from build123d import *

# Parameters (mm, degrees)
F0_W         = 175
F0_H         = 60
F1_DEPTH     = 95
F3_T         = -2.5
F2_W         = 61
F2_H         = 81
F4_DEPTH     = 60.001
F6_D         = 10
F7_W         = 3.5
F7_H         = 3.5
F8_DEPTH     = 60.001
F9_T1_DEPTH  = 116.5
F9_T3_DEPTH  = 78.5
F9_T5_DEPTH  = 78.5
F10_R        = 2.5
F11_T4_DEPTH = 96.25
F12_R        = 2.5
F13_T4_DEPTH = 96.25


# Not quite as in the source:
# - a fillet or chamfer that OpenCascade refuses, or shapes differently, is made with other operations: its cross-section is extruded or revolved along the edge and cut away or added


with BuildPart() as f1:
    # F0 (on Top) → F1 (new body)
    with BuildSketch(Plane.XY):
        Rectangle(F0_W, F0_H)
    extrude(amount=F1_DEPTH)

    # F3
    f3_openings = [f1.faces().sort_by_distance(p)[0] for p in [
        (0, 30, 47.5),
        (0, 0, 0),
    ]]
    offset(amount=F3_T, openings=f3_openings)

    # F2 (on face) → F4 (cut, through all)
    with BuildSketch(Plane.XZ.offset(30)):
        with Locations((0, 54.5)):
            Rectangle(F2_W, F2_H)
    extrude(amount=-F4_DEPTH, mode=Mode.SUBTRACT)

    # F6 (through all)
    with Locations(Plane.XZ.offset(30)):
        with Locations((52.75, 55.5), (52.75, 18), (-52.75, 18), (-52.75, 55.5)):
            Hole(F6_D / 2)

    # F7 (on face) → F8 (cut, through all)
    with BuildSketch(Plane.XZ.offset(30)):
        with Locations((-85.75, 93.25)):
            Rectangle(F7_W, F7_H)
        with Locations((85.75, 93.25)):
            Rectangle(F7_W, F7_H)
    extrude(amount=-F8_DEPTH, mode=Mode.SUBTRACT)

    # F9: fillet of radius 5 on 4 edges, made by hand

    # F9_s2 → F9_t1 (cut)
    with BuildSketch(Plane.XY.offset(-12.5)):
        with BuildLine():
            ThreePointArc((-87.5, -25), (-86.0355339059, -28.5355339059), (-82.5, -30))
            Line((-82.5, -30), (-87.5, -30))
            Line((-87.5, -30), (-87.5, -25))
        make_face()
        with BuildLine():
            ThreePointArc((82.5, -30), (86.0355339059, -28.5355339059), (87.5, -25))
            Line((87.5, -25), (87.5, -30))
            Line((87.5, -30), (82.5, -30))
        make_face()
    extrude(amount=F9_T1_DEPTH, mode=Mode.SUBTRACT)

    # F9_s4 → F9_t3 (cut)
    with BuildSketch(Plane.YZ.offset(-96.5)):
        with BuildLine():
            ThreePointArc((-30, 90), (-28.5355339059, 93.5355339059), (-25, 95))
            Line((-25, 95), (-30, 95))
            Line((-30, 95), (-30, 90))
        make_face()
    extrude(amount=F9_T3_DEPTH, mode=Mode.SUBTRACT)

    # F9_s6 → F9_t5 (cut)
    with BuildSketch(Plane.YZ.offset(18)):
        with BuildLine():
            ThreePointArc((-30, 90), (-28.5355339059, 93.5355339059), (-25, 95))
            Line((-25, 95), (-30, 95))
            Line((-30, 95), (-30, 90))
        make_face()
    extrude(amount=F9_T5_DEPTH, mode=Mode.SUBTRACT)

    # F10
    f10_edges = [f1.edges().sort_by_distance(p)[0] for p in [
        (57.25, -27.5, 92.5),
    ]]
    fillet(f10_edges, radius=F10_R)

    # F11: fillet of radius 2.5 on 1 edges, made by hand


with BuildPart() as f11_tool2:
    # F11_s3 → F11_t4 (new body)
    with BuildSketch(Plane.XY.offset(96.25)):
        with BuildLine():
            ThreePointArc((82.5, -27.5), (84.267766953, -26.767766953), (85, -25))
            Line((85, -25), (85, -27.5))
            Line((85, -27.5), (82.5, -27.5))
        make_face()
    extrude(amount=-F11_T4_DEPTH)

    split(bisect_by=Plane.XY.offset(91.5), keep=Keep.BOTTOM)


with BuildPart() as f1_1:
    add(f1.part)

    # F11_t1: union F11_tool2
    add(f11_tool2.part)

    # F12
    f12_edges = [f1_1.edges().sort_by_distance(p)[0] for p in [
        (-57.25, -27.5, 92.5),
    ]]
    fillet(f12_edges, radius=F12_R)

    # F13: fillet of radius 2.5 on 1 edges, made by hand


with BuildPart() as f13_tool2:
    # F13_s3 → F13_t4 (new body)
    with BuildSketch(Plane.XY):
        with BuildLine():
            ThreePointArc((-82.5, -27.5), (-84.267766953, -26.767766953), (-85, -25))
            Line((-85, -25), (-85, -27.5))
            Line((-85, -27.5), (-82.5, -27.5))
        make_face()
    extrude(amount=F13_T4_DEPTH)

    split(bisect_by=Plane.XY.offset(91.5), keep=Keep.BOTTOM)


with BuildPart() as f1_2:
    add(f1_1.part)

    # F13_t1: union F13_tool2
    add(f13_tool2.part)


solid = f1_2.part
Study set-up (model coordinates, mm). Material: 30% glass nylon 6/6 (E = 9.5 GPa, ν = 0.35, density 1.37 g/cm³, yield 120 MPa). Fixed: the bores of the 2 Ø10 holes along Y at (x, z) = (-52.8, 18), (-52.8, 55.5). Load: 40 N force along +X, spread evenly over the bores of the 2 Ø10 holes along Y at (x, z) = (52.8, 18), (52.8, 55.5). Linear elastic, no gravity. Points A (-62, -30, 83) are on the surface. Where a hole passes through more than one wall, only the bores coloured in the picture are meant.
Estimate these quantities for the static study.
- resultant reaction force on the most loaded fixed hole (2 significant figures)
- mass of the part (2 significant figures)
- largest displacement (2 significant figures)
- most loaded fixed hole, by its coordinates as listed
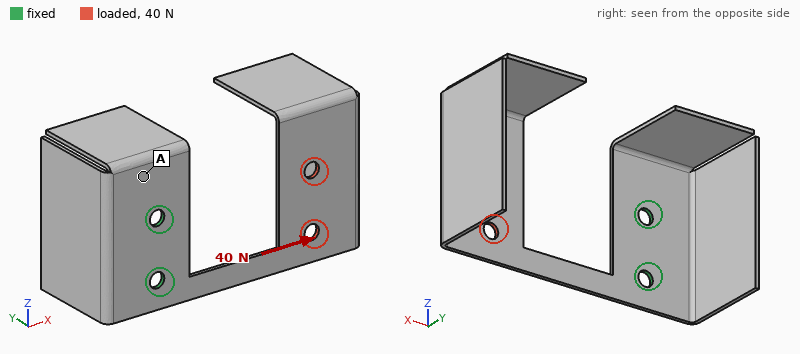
28 N
94 g
2.0 mm
(-52.8, 18)
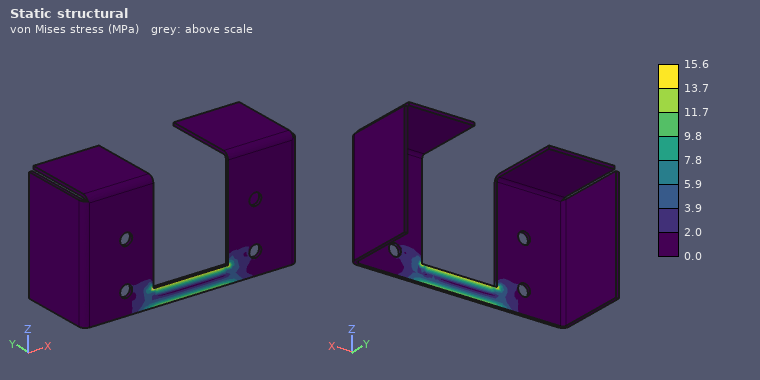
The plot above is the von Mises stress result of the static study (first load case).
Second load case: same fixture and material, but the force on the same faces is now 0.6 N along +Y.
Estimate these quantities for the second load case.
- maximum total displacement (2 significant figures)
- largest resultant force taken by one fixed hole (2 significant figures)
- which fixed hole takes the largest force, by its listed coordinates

2.2 mm
0.75 N
(-52.8, 18)
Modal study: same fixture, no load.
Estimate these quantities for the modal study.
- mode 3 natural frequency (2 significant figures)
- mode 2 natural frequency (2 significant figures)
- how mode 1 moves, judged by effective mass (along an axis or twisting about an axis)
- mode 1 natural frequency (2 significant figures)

75 Hz
28 Hz
along Y
12 Hz
